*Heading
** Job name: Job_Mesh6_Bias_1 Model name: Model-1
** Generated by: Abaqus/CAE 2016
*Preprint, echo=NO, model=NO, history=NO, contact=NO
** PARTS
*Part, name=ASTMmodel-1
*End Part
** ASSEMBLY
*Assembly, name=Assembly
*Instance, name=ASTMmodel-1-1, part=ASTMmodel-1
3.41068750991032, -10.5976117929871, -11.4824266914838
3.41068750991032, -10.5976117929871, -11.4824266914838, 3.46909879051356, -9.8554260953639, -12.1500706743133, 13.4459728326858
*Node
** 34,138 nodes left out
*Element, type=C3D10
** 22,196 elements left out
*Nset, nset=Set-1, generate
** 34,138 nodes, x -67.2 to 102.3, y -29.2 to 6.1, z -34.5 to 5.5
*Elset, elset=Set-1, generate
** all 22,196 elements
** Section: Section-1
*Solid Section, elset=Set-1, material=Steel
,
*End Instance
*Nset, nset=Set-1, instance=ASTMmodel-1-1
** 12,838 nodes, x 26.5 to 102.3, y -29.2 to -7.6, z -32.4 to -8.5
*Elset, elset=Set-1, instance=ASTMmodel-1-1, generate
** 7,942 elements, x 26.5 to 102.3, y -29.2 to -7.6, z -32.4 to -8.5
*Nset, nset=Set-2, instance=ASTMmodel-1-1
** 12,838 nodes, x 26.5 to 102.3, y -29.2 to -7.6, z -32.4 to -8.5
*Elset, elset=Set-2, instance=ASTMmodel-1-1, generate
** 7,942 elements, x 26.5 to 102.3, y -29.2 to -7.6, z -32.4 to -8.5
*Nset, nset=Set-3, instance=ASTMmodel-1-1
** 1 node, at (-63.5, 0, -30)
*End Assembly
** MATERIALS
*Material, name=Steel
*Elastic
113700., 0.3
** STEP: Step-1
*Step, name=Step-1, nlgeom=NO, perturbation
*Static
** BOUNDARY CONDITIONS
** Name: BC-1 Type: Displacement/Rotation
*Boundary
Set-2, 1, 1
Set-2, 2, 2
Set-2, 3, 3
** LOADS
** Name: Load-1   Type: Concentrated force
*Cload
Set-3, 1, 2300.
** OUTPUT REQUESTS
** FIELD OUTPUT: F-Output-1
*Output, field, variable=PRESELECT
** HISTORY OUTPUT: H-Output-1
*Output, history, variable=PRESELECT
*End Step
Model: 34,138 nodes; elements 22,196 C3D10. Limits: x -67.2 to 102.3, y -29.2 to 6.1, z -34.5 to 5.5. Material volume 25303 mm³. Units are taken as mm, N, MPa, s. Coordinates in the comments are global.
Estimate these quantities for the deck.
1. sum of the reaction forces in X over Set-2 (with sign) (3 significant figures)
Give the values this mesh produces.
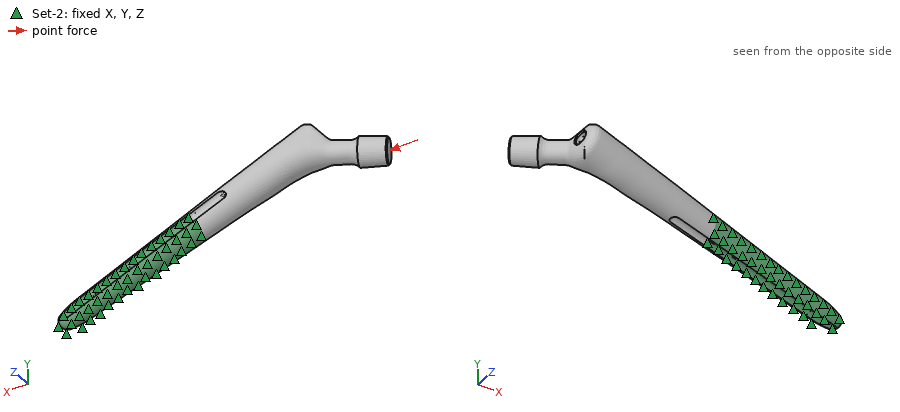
-2300 N
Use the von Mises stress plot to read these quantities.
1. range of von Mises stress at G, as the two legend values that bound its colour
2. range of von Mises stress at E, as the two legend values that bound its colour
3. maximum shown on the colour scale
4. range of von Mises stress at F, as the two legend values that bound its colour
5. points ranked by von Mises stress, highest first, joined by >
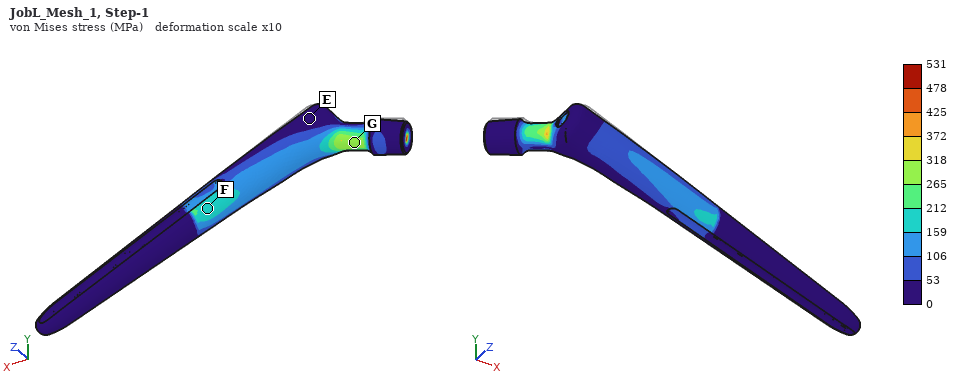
265 to 318 MPa
0 to 53 MPa
531 MPa
159 to 212 MPa
G > F > E
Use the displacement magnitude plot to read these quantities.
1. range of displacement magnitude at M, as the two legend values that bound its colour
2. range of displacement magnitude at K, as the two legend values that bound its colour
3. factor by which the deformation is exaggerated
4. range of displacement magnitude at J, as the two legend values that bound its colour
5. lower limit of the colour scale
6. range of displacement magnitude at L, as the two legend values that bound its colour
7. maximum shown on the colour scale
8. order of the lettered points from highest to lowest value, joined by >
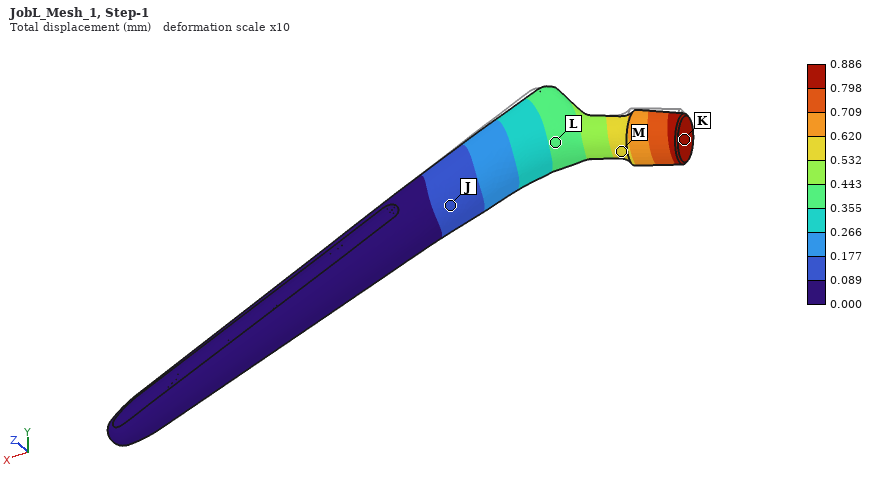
0.532 to 0.620 mm
0.798 to 0.886 mm
10
0.089 to 0.177 mm
0.000 mm
0.355 to 0.443 mm
0.886 mm
K > M > L > J
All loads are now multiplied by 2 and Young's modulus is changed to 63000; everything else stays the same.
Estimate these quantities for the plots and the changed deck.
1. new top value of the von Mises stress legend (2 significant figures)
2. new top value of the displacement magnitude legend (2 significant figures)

1100 MPa
3.2 mm
